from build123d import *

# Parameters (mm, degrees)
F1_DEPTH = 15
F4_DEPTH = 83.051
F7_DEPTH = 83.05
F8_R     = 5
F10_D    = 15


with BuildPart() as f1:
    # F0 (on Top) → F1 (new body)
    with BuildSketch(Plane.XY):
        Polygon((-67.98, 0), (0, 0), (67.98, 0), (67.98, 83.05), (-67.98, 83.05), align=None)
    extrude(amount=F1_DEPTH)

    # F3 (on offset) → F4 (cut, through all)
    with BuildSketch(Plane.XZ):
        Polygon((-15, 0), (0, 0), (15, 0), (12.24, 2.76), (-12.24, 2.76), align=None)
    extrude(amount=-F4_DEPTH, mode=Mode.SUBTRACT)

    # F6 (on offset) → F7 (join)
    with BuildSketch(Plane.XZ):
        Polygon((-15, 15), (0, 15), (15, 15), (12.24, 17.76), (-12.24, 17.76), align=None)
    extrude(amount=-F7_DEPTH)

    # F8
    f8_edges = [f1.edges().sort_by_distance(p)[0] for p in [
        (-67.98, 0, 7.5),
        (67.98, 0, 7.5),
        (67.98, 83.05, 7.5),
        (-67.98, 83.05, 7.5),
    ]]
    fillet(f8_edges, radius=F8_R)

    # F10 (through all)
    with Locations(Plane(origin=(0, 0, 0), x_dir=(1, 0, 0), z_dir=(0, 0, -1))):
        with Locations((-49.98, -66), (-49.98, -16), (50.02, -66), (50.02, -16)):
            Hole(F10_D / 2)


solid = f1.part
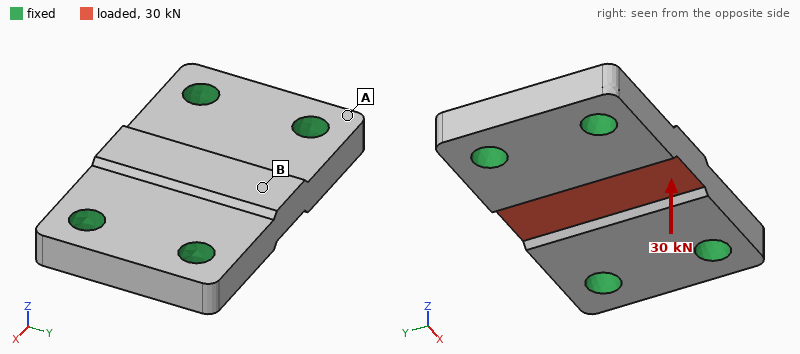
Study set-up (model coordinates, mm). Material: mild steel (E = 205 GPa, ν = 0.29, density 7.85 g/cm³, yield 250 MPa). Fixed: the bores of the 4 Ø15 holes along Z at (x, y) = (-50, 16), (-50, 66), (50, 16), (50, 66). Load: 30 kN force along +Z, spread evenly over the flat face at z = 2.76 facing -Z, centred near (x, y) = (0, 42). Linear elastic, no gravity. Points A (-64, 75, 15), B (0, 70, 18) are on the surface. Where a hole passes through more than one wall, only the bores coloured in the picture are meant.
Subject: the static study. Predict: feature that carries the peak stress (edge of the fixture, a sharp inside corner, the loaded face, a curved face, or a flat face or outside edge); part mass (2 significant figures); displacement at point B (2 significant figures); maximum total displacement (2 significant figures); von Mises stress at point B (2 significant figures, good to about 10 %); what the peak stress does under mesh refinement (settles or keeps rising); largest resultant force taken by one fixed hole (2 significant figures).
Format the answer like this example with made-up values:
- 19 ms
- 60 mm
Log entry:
- edge of the fixture
- 1.2 kg
- 30 µm
- 33 µm
- 79 MPa
- keeps rising
- 8.6 kN
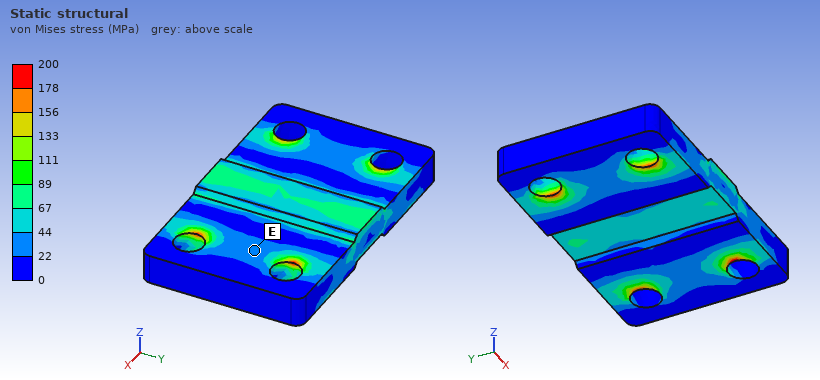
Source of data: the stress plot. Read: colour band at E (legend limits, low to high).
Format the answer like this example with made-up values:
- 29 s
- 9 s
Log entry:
- 22 to 44 MPa
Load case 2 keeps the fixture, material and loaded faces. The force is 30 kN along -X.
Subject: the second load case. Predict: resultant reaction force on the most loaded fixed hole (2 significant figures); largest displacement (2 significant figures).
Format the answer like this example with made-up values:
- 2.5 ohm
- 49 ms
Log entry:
- 7.7 kN
- 4.2 µm
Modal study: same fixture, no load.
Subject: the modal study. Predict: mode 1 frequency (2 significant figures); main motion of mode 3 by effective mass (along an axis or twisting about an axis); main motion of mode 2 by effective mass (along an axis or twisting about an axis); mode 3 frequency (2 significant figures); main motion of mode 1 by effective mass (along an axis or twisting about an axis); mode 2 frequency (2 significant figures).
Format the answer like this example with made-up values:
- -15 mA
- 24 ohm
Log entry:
- 7800 Hz
- along Y
- twisting about X
- 15 kHz
- along Z
- 9500 Hz
